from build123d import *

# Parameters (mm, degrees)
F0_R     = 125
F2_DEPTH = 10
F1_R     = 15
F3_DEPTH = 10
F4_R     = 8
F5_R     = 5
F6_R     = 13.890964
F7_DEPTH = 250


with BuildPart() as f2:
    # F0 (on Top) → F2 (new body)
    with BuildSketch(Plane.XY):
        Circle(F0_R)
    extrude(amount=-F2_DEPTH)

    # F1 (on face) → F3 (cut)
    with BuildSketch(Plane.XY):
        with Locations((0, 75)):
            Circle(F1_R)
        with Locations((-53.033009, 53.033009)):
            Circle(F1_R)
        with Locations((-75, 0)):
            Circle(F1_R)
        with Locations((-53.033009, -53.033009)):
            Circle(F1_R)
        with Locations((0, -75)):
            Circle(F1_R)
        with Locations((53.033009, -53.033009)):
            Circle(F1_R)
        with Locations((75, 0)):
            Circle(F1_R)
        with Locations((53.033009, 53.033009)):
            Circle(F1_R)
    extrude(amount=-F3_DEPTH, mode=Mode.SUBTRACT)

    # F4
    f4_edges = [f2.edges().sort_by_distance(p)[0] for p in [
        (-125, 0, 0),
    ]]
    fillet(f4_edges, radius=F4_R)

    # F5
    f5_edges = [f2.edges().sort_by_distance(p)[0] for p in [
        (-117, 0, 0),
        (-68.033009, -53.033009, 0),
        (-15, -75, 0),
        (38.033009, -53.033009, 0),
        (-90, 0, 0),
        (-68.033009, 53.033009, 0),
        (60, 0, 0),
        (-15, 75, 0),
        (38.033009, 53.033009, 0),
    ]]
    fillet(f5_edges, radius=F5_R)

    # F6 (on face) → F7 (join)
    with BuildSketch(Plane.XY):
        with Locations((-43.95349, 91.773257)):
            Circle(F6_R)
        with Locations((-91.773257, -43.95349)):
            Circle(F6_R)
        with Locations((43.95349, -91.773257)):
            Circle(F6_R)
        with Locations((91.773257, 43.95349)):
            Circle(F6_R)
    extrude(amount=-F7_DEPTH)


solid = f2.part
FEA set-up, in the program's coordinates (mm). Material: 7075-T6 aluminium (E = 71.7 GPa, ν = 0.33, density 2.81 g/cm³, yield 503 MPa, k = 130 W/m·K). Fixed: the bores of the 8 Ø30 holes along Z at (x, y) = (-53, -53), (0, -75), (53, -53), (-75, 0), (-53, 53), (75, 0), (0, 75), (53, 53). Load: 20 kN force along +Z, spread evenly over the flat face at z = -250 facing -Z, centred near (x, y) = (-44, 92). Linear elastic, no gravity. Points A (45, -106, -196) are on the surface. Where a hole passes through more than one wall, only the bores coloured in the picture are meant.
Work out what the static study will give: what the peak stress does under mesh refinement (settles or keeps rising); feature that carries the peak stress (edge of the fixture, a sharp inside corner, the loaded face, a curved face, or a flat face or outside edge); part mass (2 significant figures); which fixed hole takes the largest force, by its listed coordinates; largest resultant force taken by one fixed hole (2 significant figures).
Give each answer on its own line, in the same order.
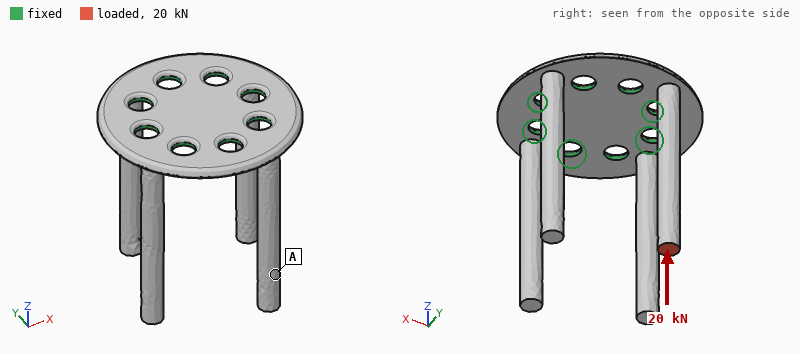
keeps rising
edge of the fixture
2.8 kg
(-53, 53)
13 kN
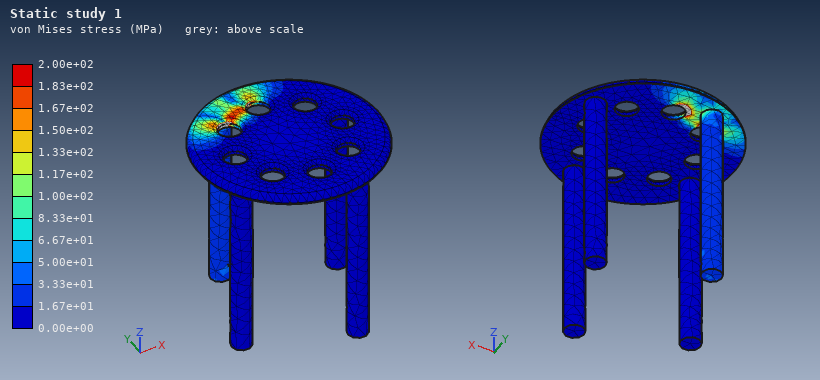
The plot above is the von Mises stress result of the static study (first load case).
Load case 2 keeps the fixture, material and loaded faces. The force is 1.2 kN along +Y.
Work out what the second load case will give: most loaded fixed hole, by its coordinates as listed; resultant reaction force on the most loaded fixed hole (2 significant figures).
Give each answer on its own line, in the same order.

(0, 75)
3.7 kN
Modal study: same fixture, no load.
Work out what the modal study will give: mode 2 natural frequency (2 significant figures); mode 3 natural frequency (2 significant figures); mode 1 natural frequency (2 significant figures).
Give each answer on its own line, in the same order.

220 Hz
220 Hz
220 Hz
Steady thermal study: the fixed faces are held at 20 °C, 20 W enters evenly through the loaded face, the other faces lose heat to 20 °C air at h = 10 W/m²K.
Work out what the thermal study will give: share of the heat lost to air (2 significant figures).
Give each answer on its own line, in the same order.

29 %
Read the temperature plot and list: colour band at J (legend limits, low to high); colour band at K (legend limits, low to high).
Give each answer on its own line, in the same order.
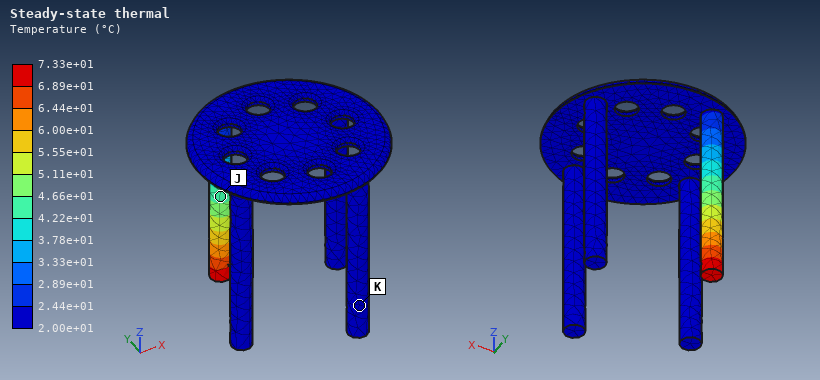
4.22e+01 to 4.66e+01 °C
2.00e+01 to 2.44e+01 °C
